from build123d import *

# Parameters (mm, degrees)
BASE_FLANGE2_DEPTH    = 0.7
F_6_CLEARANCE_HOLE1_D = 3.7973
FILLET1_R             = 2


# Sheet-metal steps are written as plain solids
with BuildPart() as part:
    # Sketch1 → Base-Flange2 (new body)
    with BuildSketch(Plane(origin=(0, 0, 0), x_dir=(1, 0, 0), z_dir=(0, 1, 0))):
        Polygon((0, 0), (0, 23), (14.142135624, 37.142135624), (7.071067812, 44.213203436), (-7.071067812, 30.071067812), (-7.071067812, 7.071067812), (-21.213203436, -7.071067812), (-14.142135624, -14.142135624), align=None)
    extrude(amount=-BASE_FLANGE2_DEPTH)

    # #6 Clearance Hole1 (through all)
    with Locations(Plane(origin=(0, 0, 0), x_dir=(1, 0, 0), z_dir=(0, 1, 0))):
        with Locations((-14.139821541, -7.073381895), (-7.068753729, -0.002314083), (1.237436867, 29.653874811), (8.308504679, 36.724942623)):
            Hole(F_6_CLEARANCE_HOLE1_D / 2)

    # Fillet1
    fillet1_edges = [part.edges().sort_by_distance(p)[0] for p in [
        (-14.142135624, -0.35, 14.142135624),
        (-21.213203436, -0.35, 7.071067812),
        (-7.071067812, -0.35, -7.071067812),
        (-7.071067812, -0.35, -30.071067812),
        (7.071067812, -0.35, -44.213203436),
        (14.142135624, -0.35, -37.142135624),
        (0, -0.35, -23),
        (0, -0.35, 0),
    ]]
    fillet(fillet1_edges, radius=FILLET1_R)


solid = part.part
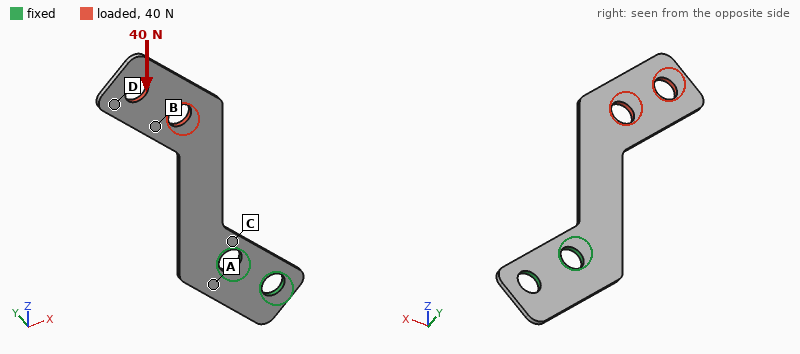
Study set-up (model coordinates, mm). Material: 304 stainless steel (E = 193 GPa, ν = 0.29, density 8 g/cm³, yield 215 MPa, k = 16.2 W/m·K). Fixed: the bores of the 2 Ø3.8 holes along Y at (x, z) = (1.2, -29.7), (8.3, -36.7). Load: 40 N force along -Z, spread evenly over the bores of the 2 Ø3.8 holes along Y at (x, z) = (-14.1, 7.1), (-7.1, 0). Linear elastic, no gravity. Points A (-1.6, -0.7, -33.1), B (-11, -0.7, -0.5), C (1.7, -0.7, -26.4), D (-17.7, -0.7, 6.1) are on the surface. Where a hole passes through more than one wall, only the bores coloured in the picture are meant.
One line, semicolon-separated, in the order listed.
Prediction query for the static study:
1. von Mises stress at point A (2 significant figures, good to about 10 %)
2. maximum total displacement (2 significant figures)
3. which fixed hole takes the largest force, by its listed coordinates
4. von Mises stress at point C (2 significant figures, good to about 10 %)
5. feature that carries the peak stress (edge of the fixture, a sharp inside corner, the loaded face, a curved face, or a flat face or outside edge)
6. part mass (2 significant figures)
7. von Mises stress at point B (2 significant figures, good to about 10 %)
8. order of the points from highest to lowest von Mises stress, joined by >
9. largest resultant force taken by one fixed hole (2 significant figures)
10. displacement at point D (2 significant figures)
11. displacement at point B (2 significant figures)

18 MPa; 62 µm; (1.2, -29.7); 26 MPa; a curved face; 2.9 g; 9.8 MPa; C > A > B > D; 47 N; 53 µm; 35 µm
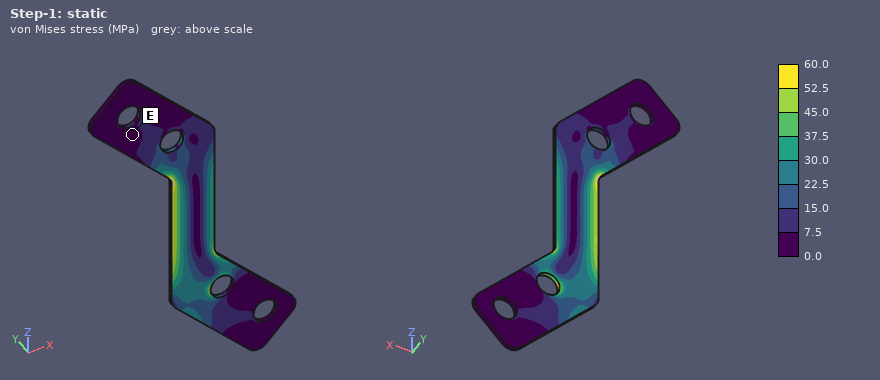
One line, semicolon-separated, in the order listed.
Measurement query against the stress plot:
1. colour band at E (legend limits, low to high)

0.0 to 7.5 MPa
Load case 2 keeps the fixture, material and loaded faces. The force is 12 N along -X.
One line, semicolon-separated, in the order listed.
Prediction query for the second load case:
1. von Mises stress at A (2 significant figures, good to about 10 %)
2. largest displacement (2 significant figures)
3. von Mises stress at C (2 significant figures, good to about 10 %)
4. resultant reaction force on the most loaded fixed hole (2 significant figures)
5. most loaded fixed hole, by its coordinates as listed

15 MPa; 52 µm; 30 MPa; 31 N; (1.2, -29.7)
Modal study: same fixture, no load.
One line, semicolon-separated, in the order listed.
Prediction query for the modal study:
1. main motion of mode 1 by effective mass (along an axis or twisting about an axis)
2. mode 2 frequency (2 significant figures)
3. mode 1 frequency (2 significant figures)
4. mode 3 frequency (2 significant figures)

along Y; 1400 Hz; 270 Hz; 2500 Hz
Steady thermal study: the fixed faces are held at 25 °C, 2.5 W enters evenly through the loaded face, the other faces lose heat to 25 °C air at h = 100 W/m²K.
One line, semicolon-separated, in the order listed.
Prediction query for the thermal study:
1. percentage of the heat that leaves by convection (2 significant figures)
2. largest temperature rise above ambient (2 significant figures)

99 %; 72 K
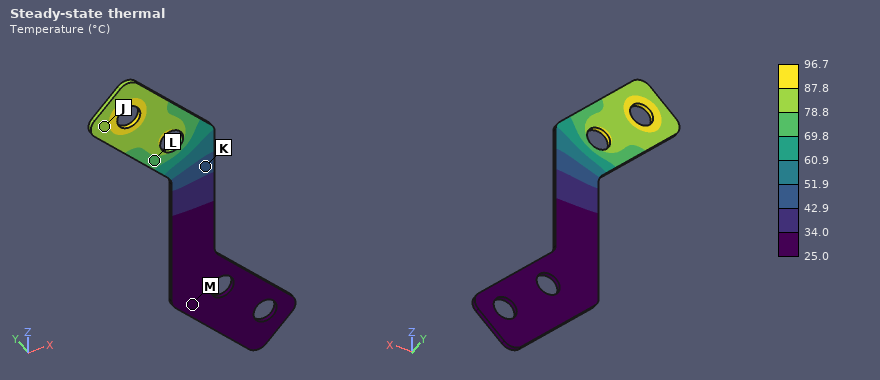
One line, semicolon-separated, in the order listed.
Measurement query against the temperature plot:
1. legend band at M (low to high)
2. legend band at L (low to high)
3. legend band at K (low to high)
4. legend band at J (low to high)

25.0 to 34.0 °C; 69.8 to 78.8 °C; 42.9 to 51.9 °C; 78.8 to 87.8 °C
